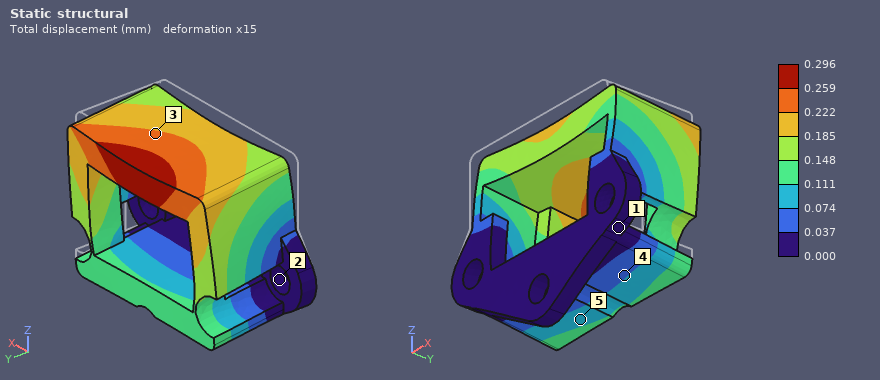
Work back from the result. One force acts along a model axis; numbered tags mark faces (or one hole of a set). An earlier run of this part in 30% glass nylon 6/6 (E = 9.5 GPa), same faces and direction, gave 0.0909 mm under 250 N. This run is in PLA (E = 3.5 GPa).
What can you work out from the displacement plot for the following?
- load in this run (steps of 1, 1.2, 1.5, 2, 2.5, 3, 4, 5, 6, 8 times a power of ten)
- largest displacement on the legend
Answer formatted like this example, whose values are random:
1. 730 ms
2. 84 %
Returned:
1. 300 N
2. 0.296 mm
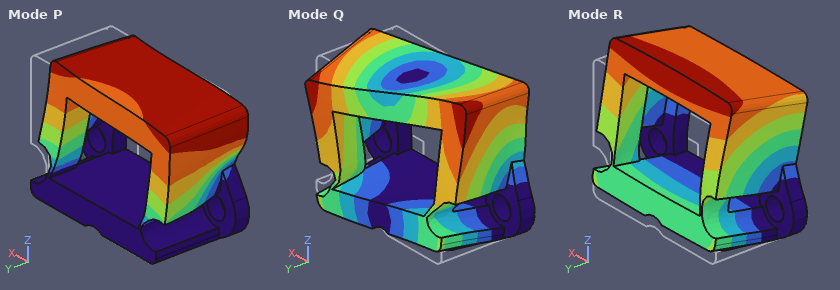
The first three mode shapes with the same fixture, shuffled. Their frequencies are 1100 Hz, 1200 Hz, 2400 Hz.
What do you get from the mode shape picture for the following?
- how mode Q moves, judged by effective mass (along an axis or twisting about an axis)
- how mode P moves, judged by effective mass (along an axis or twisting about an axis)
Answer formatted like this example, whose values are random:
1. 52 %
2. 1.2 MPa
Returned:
1. twisting about Z
2. along X
